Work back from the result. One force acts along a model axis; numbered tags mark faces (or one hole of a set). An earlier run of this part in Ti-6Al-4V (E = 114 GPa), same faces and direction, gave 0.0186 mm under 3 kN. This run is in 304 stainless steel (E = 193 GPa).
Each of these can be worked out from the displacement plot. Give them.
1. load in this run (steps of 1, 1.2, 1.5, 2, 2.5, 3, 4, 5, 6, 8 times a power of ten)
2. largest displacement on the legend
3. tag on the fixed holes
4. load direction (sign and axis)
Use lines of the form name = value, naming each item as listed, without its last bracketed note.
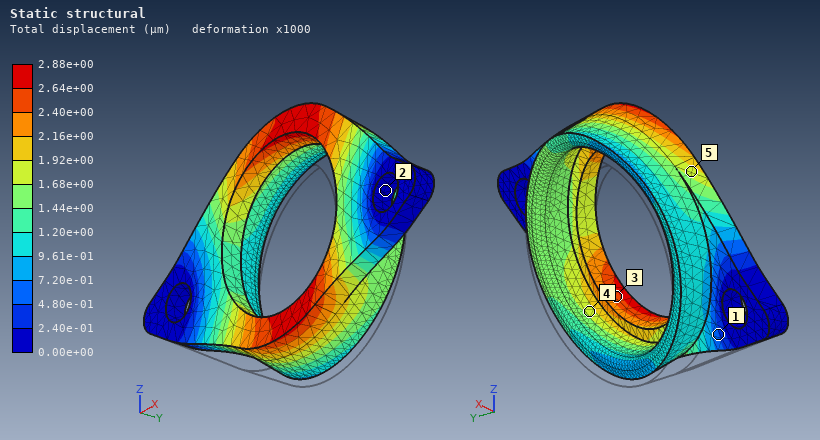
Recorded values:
load in this run = 800 N
largest displacement on the legend = 2.88e+00 µm
tag on the fixed holes = 2
load direction = +Z
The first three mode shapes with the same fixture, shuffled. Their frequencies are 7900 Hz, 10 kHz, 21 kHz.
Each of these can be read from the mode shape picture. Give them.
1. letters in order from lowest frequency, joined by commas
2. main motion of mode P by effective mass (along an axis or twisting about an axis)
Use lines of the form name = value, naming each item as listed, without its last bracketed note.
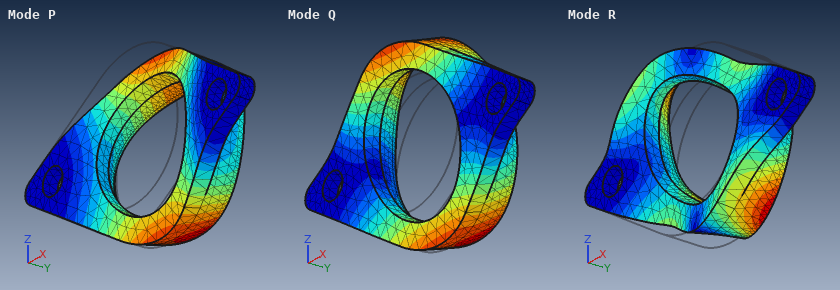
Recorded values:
letters in order from lowest frequency, joined by commas = Q, P, R
main motion of mode P by effective mass = along Y
